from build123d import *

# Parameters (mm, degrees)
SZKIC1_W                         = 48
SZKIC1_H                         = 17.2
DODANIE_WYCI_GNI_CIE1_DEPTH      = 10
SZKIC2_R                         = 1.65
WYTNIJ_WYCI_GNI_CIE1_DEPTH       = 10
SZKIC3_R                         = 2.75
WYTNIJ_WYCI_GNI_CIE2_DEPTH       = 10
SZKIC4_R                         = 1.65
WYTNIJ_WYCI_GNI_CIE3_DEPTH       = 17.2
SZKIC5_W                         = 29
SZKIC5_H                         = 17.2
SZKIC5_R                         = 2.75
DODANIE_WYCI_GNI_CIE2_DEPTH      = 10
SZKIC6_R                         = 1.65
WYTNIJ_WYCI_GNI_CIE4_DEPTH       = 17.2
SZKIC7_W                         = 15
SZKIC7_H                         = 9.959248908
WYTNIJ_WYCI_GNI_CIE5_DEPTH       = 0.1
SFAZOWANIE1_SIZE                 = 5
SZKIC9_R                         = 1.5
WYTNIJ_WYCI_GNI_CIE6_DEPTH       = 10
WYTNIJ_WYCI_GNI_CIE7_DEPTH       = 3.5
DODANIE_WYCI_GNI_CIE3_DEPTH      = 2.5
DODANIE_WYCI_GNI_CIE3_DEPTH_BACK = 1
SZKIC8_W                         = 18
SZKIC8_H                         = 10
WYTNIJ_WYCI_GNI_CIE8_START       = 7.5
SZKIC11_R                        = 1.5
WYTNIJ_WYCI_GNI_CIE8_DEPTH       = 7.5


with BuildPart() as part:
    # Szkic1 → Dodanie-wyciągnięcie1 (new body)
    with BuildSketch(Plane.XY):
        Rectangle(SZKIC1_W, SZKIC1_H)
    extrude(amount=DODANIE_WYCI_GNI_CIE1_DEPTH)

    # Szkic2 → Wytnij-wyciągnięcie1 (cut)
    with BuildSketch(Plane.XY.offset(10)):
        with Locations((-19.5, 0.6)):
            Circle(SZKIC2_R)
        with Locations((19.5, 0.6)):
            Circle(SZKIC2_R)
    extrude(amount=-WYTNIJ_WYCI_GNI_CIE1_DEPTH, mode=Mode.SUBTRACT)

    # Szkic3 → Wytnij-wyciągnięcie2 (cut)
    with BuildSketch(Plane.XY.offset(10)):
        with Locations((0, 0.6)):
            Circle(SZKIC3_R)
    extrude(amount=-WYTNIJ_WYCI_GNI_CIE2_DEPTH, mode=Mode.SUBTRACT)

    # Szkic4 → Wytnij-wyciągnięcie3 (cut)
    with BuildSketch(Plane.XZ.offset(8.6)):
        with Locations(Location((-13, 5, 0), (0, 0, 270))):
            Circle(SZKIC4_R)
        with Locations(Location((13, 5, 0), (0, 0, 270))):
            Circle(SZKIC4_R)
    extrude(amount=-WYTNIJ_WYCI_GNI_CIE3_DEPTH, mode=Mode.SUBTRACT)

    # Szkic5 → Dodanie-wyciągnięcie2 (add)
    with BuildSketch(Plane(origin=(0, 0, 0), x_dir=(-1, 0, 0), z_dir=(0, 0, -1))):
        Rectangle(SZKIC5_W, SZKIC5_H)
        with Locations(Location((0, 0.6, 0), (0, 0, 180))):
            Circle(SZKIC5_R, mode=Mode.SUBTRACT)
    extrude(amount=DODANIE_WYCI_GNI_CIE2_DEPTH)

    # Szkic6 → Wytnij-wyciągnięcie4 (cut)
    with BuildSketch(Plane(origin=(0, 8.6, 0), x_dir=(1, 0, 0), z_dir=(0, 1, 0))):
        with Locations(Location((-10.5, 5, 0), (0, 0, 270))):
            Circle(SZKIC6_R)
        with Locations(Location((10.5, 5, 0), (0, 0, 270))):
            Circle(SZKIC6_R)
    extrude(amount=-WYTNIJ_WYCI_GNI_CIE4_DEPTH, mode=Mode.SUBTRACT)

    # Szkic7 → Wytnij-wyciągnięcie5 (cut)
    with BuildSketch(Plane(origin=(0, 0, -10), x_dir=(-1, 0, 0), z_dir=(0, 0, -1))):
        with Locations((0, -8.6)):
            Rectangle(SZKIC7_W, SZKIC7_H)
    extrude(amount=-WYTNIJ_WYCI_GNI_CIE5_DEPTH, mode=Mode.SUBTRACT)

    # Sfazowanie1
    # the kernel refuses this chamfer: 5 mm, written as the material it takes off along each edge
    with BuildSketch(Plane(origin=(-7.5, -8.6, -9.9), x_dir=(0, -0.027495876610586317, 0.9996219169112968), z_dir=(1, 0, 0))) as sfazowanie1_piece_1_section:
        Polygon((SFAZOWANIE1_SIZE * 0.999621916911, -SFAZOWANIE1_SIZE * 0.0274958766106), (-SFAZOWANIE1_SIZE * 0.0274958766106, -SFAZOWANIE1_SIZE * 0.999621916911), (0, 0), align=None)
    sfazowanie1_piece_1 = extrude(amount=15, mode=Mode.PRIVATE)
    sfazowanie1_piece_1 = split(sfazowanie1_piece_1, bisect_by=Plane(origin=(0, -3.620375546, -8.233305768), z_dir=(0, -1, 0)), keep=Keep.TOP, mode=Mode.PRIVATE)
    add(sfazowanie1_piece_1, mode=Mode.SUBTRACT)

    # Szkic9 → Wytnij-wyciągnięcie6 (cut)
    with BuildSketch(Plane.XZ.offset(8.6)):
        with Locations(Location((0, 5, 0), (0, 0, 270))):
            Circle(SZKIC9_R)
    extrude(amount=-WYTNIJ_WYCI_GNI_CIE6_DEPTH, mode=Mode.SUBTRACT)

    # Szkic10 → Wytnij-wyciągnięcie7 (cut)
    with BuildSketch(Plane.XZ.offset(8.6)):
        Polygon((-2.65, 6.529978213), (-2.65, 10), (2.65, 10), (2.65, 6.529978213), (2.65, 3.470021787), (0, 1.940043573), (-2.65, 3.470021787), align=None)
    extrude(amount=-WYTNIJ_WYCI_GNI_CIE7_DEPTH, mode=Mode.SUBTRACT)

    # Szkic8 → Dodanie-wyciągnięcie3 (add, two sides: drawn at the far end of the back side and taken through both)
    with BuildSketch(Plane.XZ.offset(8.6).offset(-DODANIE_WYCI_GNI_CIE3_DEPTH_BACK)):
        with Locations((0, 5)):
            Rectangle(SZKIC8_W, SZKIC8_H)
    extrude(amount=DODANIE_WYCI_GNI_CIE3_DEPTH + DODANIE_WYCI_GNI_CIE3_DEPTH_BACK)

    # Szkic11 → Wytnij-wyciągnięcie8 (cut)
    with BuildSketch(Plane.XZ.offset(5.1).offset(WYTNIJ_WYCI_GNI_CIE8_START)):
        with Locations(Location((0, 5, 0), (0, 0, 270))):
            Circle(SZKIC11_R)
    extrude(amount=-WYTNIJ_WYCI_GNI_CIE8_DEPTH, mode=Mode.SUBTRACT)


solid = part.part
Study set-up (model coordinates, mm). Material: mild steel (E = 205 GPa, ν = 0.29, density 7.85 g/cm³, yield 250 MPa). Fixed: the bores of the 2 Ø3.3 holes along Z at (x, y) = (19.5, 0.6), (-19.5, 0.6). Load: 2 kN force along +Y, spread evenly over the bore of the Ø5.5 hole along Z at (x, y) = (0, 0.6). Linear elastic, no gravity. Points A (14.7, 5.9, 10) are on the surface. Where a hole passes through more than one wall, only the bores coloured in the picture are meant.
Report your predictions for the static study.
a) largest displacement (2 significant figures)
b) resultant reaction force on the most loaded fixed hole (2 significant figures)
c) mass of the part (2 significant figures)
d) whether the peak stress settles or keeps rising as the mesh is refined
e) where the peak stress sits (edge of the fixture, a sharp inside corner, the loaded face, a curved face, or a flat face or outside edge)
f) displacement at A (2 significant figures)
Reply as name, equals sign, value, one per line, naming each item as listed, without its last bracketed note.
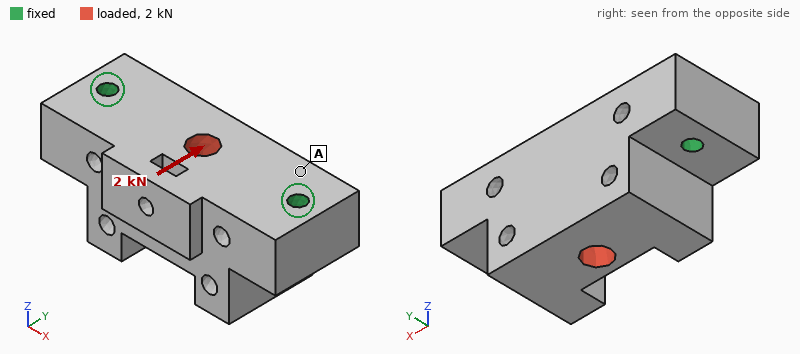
largest displacement = 5.6 µm
resultant reaction force on the most loaded fixed hole = 1.0 kN
mass of the part = 95 g
whether the peak stress settles or keeps rising as the mesh is refined = keeps rising
where the peak stress sits = edge of the fixture
displacement at A = 0.91 µm
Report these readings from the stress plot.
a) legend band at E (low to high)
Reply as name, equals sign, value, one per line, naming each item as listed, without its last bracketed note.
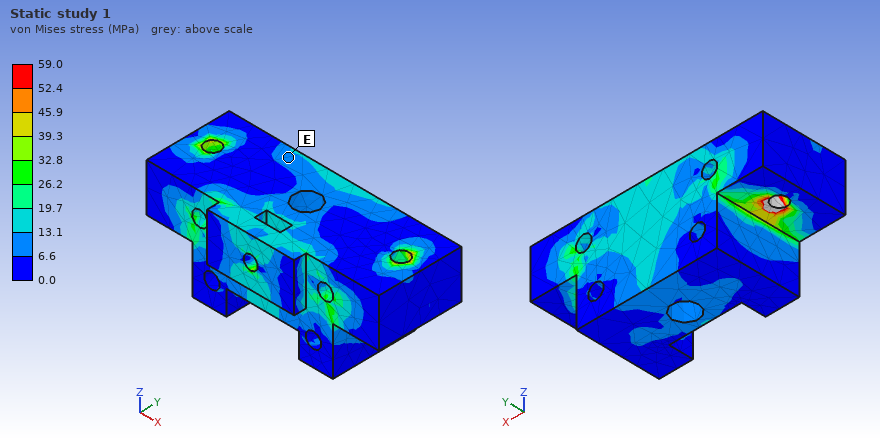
legend band at E = 6.6 to 13.1 MPa
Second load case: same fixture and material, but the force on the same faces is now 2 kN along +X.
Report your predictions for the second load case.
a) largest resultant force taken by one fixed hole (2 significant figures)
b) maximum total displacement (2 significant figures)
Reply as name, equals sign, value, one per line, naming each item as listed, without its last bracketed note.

largest resultant force taken by one fixed hole = 1.0 kN
maximum total displacement = 1.0 µm
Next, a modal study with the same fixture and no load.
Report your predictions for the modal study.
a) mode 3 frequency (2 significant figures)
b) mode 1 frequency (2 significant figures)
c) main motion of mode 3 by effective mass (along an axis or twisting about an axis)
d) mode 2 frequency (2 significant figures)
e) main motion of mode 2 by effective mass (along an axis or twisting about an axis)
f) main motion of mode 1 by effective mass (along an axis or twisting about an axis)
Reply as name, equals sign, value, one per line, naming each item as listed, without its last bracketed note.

mode 3 frequency = 25 kHz
mode 1 frequency = 14 kHz
main motion of mode 3 by effective mass = along Y
mode 2 frequency = 21 kHz
main motion of mode 2 by effective mass = along Z
main motion of mode 1 by effective mass = along Y
